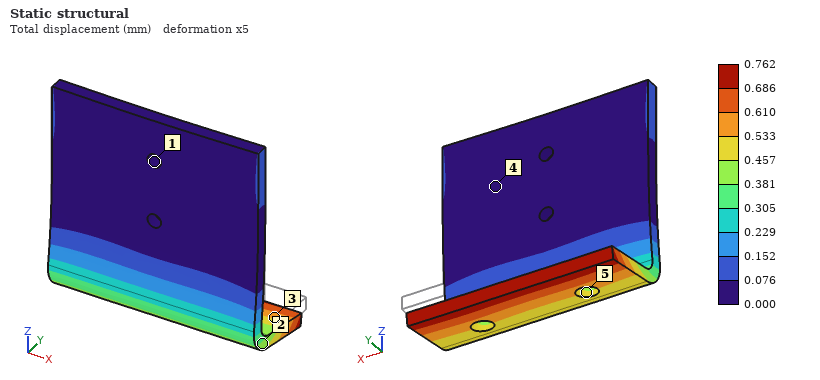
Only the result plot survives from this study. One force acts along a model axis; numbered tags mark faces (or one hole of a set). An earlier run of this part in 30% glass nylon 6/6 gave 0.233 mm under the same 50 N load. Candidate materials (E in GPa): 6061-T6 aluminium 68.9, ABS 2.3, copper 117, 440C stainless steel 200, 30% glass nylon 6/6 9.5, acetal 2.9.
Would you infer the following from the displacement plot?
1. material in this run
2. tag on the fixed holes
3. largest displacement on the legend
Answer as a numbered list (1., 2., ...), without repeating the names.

1. acetal
2. 1
3. 0.762 mm
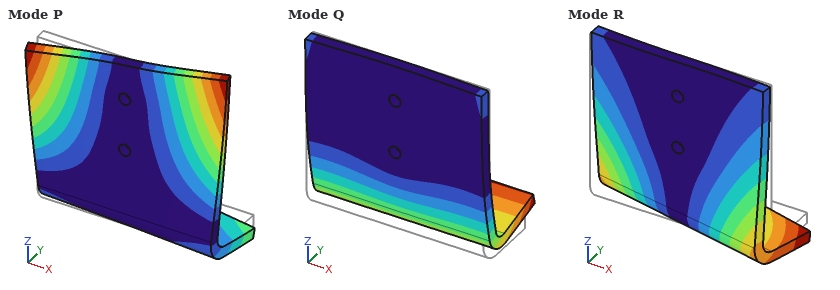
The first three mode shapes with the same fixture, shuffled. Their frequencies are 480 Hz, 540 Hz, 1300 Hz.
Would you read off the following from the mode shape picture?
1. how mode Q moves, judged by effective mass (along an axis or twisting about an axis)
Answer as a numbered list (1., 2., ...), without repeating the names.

1. along Y
